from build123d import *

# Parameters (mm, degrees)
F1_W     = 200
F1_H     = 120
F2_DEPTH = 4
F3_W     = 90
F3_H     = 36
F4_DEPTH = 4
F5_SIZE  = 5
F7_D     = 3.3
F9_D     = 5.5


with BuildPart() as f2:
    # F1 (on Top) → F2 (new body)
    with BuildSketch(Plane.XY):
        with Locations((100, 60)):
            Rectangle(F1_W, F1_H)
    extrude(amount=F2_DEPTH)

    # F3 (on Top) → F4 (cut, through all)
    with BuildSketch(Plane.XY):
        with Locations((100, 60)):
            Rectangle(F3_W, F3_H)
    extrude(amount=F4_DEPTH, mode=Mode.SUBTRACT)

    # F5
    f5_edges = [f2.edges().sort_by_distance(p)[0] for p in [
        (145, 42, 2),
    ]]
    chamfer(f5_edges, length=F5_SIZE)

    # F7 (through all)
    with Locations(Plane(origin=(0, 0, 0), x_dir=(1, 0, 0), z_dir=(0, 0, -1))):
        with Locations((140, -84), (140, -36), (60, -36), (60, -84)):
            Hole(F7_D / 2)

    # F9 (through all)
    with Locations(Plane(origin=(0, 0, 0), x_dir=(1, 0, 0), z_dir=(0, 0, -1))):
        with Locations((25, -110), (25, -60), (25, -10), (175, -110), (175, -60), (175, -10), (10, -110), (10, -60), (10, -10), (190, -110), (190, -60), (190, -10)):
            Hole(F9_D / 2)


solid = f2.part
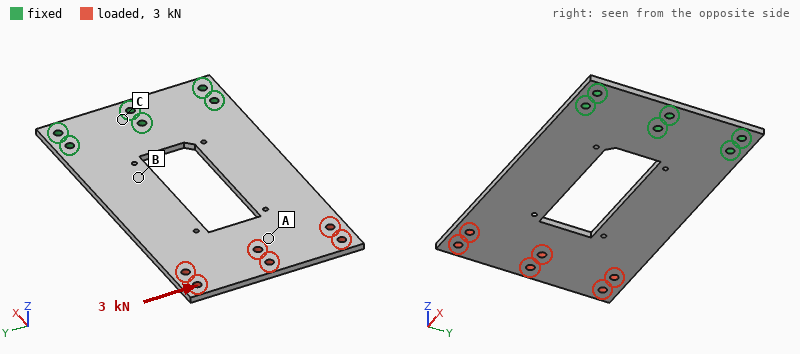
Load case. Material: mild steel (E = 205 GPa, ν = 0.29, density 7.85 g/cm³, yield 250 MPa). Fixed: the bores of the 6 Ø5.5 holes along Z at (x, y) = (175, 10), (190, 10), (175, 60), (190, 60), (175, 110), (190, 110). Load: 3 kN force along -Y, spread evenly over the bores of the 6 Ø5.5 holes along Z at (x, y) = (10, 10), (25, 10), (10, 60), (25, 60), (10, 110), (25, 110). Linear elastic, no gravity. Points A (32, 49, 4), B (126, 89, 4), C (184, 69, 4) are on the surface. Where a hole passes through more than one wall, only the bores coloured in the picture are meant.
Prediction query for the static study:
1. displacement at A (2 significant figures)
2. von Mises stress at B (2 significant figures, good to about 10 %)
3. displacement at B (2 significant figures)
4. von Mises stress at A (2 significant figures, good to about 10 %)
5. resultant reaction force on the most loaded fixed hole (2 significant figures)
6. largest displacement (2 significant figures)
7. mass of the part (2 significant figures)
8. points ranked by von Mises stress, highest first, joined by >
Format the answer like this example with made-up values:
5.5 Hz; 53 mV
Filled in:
0.093 mm; 19 MPa; 0.019 mm; 33 MPa; 3.9 kN; 0.11 mm; 640 g; A > B > C
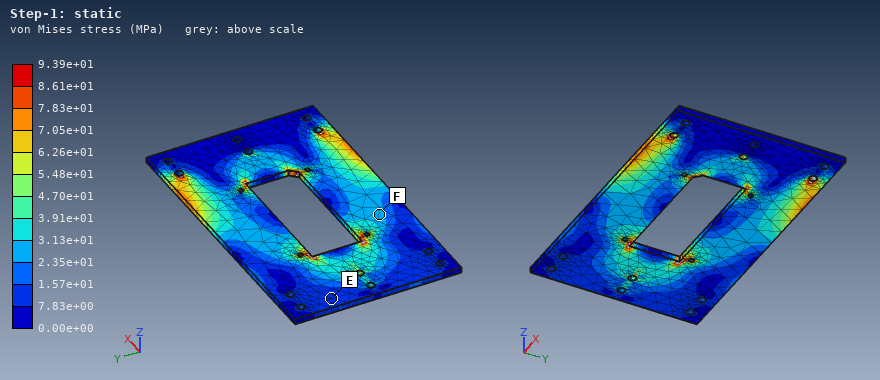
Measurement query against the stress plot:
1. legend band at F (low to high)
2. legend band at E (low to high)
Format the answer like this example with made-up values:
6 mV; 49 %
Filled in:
2.35e+01 to 3.13e+01 MPa; 7.83e+00 to 1.57e+01 MPa
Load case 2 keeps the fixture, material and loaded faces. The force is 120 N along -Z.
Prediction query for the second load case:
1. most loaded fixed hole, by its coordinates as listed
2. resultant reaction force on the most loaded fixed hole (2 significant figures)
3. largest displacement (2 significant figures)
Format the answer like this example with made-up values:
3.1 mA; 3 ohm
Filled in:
(175, 60); 290 N; 1.8 mm
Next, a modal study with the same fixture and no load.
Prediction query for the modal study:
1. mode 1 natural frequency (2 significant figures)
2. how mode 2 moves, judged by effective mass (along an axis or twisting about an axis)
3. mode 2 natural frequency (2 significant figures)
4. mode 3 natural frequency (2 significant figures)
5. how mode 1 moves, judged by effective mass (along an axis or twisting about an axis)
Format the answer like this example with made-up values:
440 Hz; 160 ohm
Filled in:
100 Hz; twisting about X; 320 Hz; 670 Hz; along Z
